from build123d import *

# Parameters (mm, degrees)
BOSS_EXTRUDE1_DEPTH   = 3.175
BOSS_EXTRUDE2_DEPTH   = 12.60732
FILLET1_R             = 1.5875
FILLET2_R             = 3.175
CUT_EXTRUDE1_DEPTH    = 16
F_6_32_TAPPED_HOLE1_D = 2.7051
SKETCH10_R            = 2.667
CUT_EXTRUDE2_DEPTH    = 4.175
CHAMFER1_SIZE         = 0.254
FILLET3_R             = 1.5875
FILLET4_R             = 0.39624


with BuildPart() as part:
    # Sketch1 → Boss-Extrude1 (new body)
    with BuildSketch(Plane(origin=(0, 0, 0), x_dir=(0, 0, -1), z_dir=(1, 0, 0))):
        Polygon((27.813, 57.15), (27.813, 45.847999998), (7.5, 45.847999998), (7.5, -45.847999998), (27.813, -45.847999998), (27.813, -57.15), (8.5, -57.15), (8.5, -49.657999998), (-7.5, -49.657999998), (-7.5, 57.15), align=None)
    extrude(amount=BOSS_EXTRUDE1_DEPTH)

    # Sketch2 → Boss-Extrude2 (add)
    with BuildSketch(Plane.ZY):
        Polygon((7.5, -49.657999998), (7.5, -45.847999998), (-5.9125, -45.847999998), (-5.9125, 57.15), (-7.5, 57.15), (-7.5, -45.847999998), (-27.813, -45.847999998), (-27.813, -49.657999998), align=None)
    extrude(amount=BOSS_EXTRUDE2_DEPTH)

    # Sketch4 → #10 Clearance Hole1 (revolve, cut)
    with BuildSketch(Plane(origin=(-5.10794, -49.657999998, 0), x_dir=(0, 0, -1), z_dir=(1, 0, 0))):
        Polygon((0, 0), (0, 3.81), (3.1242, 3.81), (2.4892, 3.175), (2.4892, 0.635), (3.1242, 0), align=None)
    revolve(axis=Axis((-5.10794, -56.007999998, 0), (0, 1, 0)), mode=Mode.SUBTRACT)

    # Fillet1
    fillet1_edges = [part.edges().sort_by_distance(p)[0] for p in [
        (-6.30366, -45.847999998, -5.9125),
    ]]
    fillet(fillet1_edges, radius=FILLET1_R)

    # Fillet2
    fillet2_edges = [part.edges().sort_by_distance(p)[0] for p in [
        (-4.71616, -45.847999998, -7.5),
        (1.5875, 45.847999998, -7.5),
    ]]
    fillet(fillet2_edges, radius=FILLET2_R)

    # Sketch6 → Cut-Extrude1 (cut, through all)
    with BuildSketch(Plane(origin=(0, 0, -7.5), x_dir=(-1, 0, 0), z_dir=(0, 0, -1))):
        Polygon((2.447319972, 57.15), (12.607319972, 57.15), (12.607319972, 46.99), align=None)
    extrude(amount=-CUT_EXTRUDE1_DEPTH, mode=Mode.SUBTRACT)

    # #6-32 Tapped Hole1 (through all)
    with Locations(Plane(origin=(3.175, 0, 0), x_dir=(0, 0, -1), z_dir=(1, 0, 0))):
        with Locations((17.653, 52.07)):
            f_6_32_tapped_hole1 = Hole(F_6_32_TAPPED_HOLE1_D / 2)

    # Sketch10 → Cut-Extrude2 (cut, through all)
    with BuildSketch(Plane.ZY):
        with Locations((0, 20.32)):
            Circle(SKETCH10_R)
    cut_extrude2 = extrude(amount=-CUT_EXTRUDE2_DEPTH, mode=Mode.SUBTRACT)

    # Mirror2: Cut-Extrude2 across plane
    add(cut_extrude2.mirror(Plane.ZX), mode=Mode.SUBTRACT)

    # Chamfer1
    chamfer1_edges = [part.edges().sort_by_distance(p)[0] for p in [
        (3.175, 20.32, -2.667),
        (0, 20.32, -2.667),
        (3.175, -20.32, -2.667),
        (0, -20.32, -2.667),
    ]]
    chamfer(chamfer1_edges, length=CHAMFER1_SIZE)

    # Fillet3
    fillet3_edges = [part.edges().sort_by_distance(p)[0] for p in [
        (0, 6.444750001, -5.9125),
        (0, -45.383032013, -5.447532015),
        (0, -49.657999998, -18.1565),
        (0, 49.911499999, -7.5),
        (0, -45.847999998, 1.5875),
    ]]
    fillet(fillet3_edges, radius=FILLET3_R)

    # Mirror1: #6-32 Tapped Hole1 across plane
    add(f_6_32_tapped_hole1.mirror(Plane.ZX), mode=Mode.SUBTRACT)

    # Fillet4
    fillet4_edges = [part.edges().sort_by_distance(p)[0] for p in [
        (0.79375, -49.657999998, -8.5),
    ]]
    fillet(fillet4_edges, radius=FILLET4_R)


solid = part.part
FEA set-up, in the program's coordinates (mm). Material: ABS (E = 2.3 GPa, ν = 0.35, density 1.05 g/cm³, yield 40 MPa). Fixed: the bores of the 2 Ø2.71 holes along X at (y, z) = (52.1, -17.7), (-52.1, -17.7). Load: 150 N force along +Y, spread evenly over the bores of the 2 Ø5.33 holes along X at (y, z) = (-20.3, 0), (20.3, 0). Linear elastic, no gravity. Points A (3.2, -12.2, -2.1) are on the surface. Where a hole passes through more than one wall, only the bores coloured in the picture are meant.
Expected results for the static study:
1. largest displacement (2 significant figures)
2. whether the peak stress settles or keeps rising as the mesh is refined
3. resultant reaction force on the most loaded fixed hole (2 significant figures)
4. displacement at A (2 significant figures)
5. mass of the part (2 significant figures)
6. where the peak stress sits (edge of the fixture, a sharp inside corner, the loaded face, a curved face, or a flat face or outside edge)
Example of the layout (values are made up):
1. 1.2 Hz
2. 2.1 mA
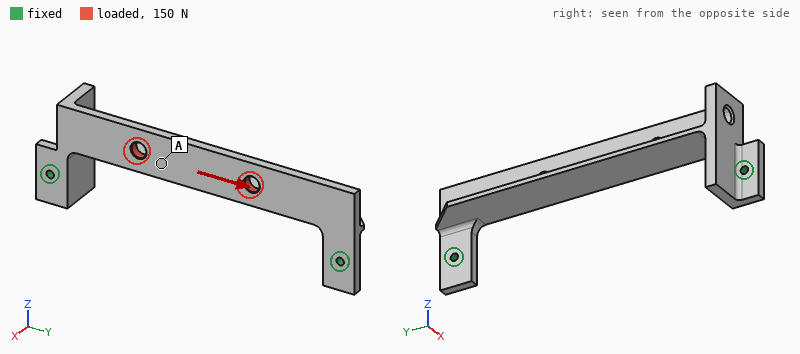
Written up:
1. 0.22 mm
2. keeps rising
3. 78 N
4. 0.16 mm
5. 11 g
6. edge of the fixture
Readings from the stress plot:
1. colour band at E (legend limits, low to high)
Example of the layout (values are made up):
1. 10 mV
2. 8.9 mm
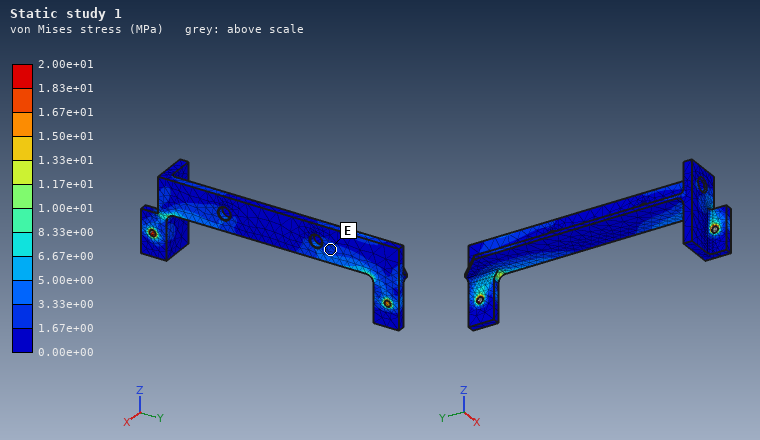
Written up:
1. 1.67e+00 to 3.33e+00 MPa
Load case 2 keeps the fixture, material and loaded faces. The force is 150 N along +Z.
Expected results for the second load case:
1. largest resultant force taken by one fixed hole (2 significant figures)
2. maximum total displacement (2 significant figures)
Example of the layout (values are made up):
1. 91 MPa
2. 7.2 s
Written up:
1. 110 N
2. 0.48 mm
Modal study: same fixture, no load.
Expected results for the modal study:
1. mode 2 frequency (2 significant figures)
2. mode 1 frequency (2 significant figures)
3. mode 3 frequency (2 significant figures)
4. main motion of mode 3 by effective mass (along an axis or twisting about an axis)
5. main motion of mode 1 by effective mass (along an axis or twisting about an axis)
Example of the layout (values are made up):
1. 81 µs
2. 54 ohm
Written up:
1. 990 Hz
2. 520 Hz
3. 1100 Hz
4. along Z
5. along X
